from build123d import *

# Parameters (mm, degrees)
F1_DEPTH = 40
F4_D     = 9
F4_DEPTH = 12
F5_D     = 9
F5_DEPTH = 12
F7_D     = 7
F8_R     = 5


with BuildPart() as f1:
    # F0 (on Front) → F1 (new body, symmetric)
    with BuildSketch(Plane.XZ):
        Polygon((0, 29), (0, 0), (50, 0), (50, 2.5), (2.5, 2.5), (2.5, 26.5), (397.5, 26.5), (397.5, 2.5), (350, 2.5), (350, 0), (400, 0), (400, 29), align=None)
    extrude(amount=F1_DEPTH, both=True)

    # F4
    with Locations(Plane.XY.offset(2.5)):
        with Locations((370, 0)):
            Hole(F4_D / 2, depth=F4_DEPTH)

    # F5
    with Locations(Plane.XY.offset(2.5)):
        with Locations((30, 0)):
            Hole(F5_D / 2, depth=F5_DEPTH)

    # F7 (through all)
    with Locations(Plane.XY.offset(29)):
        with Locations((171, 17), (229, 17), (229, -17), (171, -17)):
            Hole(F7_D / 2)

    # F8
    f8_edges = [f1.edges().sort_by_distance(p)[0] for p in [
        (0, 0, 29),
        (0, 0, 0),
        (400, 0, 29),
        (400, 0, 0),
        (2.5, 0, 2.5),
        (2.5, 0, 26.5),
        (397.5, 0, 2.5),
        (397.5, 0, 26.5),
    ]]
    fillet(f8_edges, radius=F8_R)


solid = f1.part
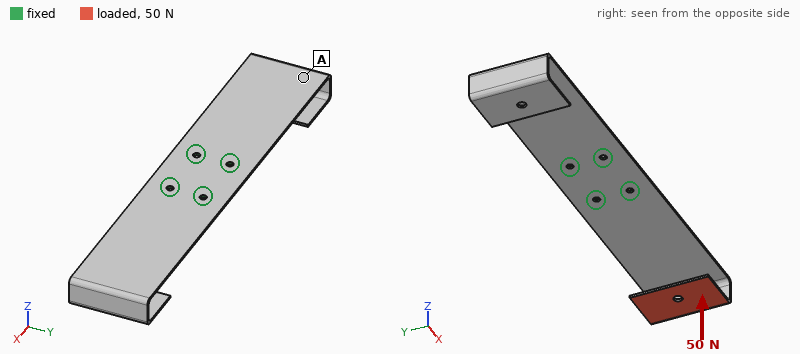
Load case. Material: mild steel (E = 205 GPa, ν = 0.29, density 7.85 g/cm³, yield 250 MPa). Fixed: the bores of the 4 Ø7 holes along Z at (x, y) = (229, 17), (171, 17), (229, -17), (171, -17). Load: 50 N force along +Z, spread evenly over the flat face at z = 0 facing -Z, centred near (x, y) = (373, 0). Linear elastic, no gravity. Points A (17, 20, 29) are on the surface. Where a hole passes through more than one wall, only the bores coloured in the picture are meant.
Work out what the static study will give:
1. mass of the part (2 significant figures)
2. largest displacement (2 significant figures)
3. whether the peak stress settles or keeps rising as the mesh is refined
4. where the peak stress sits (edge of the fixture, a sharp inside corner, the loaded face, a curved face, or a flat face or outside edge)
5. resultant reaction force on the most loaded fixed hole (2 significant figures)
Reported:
850 g
2.9 mm
keeps rising
edge of the fixture
31 N
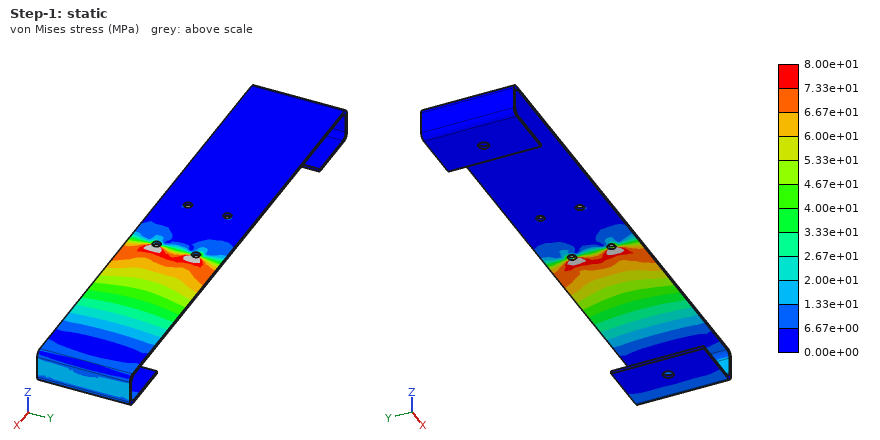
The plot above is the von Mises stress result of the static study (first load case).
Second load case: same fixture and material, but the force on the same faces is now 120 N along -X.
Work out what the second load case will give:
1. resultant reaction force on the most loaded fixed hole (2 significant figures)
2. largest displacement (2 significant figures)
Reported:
52 N
2.3 mm
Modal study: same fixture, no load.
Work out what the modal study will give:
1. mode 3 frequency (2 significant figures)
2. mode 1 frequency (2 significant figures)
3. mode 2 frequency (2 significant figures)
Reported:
180 Hz
47 Hz
47 Hz
